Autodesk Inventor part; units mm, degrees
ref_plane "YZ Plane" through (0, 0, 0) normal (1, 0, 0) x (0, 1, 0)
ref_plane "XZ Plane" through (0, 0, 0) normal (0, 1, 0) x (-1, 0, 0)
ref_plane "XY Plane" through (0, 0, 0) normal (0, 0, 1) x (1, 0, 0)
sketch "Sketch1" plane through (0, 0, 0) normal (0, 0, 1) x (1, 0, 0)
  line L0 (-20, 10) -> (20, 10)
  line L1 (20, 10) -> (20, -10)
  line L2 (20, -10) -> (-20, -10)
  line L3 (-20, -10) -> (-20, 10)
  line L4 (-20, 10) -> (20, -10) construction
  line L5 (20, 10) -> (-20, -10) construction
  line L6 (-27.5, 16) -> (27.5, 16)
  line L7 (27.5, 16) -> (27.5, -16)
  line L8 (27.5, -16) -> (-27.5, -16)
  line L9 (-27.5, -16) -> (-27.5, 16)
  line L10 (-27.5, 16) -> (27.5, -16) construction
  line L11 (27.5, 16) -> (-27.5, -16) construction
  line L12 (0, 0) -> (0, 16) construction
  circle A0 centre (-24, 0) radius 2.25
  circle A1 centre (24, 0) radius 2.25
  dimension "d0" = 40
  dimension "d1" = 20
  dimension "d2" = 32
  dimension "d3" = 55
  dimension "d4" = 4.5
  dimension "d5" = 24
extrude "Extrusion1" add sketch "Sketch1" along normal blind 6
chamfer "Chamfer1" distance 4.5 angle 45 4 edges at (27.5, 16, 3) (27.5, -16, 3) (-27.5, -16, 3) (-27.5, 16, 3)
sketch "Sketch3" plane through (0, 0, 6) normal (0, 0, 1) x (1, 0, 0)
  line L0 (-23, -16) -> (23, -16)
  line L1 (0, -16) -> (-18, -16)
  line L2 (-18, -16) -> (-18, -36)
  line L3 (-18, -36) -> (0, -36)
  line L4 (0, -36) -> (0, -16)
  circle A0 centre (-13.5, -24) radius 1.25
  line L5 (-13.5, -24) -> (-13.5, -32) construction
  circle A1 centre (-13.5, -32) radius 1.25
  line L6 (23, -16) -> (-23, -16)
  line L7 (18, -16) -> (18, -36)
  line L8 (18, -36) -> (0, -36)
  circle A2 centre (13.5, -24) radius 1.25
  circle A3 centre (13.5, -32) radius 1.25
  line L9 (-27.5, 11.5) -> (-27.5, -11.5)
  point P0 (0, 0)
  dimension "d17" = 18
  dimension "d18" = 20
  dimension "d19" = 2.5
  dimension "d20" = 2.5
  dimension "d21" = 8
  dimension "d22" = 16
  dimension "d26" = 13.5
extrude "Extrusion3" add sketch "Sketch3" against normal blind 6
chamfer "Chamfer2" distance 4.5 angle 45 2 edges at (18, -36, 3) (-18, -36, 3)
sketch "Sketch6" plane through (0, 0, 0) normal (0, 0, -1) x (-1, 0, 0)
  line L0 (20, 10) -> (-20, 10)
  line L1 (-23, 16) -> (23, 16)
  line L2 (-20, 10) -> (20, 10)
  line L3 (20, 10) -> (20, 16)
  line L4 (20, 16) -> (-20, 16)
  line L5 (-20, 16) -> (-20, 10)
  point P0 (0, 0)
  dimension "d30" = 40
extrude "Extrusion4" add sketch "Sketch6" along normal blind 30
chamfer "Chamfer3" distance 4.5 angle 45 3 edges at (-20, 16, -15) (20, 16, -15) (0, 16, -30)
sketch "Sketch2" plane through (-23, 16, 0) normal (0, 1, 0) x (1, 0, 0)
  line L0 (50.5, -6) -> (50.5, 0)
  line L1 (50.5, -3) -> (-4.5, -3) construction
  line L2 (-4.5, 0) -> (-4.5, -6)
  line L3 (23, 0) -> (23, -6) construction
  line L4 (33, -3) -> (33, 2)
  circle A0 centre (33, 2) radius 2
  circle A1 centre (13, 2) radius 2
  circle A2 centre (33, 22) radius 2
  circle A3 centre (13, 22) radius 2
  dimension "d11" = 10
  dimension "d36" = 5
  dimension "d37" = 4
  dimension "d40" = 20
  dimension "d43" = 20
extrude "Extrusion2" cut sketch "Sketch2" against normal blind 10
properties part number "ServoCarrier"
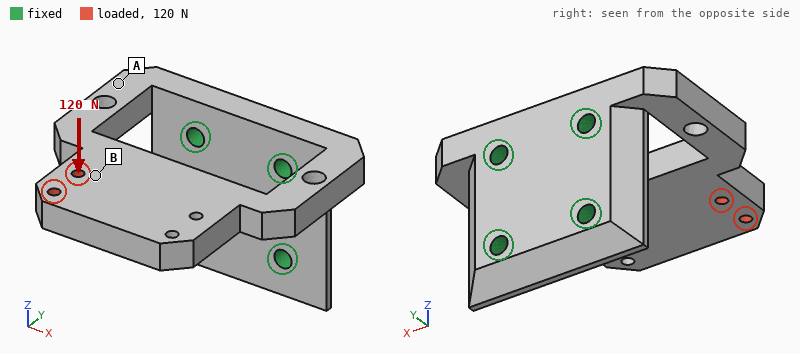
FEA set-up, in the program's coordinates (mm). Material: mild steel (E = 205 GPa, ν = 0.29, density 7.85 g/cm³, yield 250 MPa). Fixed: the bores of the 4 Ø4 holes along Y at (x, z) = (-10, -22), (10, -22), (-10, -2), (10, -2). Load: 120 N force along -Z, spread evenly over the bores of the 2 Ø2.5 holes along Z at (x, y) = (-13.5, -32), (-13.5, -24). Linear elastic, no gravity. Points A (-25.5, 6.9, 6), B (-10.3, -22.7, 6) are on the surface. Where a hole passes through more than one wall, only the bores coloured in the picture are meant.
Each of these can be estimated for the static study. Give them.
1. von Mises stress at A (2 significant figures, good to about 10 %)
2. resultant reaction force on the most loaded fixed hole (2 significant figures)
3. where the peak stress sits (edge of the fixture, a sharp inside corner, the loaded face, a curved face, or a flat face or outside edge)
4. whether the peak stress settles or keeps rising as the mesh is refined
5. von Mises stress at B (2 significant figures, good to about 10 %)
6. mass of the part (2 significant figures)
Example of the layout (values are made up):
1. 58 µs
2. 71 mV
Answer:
1. 46 MPa
2. 92 N
3. a sharp inside corner
4. keeps rising
5. 13 MPa
6. 120 g
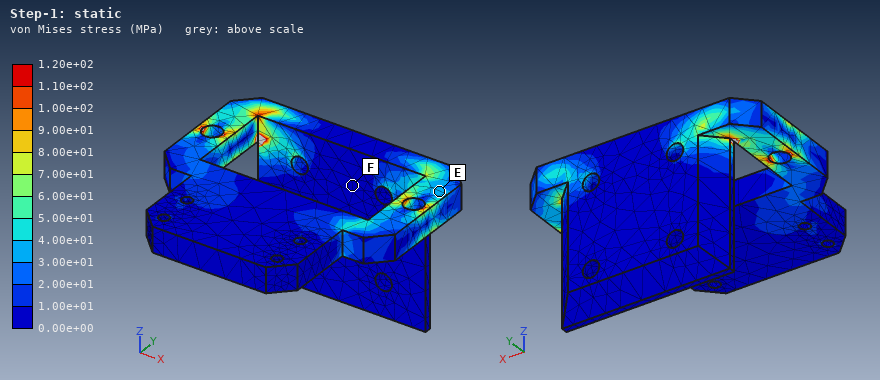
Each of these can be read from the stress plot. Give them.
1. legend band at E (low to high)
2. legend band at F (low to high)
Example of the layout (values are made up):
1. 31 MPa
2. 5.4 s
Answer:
1. 3.00e+01 to 4.00e+01 MPa
2. 0.00e+00 to 1.00e+01 MPa
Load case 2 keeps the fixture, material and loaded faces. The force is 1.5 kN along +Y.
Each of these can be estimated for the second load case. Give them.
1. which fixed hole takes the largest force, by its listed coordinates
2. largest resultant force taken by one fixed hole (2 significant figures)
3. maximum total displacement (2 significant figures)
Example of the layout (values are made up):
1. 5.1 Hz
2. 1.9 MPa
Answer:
1. (-10, -2)
2. 1.4 kN
3. 51 µm
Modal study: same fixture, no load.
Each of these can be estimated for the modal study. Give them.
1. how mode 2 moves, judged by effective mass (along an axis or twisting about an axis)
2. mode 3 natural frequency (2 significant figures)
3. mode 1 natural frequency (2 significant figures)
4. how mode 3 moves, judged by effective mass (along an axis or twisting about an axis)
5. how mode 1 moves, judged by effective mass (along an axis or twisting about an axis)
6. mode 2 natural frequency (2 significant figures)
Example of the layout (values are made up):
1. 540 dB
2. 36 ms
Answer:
1. along X
2. 3700 Hz
3. 900 Hz
4. twisting about Y
5. along Z
6. 2000 Hz
